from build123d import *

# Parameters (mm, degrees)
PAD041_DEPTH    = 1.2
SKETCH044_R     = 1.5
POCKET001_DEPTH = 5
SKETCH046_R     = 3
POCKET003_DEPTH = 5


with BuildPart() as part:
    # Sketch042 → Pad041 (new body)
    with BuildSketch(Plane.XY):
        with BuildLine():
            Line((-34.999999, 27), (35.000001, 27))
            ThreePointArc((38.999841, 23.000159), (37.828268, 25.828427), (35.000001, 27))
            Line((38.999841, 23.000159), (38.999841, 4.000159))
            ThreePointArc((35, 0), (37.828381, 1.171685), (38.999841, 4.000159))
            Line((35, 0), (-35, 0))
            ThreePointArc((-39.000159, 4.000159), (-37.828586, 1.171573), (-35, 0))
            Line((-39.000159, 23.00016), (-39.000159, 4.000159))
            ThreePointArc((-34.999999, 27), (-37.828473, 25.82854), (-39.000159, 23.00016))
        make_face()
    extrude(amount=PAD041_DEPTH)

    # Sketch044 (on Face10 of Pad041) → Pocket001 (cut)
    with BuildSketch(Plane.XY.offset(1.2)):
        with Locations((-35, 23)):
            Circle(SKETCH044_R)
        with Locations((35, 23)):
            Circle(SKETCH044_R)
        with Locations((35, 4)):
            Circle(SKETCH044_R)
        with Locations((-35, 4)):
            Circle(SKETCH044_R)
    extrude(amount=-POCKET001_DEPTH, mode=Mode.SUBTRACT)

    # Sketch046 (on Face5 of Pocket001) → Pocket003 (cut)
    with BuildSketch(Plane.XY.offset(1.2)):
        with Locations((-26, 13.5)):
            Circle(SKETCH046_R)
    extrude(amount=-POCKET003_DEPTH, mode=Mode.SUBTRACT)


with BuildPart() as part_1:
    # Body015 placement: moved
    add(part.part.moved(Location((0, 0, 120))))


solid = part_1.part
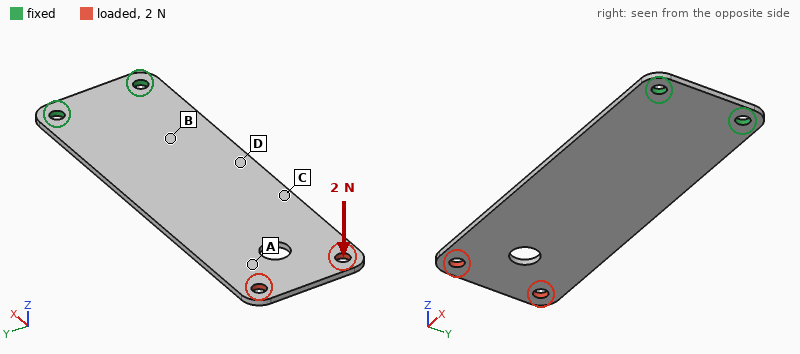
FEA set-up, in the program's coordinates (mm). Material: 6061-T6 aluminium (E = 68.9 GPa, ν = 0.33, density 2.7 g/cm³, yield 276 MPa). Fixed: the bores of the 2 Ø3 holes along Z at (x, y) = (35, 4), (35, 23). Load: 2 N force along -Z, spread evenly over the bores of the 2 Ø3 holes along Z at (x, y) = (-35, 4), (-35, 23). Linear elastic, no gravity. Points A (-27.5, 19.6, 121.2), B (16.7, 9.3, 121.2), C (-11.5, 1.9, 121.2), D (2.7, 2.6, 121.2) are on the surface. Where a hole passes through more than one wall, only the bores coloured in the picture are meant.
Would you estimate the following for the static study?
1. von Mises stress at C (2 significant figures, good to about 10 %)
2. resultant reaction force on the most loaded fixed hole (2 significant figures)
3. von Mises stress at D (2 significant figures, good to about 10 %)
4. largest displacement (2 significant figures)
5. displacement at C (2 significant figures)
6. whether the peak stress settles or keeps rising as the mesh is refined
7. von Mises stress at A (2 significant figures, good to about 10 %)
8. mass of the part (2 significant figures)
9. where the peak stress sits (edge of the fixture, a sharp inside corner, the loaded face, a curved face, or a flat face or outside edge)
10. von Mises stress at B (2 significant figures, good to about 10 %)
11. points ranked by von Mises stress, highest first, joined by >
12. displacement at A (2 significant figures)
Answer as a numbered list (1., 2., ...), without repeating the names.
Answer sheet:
1. 7.4 MPa
2. 1.0 N
3. 12 MPa
4. 0.90 mm
5. 0.42 mm
6. keeps rising
7. 3.1 MPa
8. 6.6 g
9. edge of the fixture
10. 15 MPa
11. B > D > C > A
12. 0.70 mm
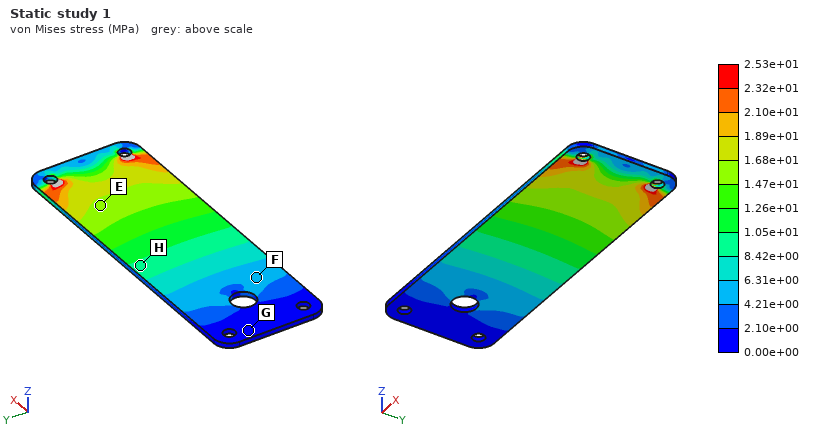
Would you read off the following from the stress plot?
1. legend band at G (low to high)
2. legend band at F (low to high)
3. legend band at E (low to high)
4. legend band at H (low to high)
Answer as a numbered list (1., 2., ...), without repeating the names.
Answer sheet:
1. 0.00e+00 to 2.10e+00 MPa
2. 4.21e+00 to 6.31e+00 MPa
3. 1.47e+01 to 1.68e+01 MPa
4. 8.42e+00 to 1.05e+01 MPa
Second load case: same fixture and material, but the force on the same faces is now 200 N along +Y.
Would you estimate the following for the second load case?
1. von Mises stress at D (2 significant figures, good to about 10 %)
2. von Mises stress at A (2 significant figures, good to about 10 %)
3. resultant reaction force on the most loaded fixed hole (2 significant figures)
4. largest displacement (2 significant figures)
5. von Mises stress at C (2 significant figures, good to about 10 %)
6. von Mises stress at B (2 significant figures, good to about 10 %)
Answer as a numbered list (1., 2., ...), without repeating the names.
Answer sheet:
1. 42 MPa
2. 19 MPa
3. 700 N
4. 0.21 mm
5. 29 MPa
6. 27 MPa
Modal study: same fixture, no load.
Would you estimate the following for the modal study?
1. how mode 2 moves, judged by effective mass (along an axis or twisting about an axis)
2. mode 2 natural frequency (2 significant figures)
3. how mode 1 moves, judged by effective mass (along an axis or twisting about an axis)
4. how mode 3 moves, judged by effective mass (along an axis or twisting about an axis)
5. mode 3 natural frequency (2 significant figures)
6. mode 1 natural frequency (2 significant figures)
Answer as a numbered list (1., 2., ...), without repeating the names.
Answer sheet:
1. twisting about X
2. 1000 Hz
3. along Z
4. along Z
5. 1200 Hz
6. 190 Hz
